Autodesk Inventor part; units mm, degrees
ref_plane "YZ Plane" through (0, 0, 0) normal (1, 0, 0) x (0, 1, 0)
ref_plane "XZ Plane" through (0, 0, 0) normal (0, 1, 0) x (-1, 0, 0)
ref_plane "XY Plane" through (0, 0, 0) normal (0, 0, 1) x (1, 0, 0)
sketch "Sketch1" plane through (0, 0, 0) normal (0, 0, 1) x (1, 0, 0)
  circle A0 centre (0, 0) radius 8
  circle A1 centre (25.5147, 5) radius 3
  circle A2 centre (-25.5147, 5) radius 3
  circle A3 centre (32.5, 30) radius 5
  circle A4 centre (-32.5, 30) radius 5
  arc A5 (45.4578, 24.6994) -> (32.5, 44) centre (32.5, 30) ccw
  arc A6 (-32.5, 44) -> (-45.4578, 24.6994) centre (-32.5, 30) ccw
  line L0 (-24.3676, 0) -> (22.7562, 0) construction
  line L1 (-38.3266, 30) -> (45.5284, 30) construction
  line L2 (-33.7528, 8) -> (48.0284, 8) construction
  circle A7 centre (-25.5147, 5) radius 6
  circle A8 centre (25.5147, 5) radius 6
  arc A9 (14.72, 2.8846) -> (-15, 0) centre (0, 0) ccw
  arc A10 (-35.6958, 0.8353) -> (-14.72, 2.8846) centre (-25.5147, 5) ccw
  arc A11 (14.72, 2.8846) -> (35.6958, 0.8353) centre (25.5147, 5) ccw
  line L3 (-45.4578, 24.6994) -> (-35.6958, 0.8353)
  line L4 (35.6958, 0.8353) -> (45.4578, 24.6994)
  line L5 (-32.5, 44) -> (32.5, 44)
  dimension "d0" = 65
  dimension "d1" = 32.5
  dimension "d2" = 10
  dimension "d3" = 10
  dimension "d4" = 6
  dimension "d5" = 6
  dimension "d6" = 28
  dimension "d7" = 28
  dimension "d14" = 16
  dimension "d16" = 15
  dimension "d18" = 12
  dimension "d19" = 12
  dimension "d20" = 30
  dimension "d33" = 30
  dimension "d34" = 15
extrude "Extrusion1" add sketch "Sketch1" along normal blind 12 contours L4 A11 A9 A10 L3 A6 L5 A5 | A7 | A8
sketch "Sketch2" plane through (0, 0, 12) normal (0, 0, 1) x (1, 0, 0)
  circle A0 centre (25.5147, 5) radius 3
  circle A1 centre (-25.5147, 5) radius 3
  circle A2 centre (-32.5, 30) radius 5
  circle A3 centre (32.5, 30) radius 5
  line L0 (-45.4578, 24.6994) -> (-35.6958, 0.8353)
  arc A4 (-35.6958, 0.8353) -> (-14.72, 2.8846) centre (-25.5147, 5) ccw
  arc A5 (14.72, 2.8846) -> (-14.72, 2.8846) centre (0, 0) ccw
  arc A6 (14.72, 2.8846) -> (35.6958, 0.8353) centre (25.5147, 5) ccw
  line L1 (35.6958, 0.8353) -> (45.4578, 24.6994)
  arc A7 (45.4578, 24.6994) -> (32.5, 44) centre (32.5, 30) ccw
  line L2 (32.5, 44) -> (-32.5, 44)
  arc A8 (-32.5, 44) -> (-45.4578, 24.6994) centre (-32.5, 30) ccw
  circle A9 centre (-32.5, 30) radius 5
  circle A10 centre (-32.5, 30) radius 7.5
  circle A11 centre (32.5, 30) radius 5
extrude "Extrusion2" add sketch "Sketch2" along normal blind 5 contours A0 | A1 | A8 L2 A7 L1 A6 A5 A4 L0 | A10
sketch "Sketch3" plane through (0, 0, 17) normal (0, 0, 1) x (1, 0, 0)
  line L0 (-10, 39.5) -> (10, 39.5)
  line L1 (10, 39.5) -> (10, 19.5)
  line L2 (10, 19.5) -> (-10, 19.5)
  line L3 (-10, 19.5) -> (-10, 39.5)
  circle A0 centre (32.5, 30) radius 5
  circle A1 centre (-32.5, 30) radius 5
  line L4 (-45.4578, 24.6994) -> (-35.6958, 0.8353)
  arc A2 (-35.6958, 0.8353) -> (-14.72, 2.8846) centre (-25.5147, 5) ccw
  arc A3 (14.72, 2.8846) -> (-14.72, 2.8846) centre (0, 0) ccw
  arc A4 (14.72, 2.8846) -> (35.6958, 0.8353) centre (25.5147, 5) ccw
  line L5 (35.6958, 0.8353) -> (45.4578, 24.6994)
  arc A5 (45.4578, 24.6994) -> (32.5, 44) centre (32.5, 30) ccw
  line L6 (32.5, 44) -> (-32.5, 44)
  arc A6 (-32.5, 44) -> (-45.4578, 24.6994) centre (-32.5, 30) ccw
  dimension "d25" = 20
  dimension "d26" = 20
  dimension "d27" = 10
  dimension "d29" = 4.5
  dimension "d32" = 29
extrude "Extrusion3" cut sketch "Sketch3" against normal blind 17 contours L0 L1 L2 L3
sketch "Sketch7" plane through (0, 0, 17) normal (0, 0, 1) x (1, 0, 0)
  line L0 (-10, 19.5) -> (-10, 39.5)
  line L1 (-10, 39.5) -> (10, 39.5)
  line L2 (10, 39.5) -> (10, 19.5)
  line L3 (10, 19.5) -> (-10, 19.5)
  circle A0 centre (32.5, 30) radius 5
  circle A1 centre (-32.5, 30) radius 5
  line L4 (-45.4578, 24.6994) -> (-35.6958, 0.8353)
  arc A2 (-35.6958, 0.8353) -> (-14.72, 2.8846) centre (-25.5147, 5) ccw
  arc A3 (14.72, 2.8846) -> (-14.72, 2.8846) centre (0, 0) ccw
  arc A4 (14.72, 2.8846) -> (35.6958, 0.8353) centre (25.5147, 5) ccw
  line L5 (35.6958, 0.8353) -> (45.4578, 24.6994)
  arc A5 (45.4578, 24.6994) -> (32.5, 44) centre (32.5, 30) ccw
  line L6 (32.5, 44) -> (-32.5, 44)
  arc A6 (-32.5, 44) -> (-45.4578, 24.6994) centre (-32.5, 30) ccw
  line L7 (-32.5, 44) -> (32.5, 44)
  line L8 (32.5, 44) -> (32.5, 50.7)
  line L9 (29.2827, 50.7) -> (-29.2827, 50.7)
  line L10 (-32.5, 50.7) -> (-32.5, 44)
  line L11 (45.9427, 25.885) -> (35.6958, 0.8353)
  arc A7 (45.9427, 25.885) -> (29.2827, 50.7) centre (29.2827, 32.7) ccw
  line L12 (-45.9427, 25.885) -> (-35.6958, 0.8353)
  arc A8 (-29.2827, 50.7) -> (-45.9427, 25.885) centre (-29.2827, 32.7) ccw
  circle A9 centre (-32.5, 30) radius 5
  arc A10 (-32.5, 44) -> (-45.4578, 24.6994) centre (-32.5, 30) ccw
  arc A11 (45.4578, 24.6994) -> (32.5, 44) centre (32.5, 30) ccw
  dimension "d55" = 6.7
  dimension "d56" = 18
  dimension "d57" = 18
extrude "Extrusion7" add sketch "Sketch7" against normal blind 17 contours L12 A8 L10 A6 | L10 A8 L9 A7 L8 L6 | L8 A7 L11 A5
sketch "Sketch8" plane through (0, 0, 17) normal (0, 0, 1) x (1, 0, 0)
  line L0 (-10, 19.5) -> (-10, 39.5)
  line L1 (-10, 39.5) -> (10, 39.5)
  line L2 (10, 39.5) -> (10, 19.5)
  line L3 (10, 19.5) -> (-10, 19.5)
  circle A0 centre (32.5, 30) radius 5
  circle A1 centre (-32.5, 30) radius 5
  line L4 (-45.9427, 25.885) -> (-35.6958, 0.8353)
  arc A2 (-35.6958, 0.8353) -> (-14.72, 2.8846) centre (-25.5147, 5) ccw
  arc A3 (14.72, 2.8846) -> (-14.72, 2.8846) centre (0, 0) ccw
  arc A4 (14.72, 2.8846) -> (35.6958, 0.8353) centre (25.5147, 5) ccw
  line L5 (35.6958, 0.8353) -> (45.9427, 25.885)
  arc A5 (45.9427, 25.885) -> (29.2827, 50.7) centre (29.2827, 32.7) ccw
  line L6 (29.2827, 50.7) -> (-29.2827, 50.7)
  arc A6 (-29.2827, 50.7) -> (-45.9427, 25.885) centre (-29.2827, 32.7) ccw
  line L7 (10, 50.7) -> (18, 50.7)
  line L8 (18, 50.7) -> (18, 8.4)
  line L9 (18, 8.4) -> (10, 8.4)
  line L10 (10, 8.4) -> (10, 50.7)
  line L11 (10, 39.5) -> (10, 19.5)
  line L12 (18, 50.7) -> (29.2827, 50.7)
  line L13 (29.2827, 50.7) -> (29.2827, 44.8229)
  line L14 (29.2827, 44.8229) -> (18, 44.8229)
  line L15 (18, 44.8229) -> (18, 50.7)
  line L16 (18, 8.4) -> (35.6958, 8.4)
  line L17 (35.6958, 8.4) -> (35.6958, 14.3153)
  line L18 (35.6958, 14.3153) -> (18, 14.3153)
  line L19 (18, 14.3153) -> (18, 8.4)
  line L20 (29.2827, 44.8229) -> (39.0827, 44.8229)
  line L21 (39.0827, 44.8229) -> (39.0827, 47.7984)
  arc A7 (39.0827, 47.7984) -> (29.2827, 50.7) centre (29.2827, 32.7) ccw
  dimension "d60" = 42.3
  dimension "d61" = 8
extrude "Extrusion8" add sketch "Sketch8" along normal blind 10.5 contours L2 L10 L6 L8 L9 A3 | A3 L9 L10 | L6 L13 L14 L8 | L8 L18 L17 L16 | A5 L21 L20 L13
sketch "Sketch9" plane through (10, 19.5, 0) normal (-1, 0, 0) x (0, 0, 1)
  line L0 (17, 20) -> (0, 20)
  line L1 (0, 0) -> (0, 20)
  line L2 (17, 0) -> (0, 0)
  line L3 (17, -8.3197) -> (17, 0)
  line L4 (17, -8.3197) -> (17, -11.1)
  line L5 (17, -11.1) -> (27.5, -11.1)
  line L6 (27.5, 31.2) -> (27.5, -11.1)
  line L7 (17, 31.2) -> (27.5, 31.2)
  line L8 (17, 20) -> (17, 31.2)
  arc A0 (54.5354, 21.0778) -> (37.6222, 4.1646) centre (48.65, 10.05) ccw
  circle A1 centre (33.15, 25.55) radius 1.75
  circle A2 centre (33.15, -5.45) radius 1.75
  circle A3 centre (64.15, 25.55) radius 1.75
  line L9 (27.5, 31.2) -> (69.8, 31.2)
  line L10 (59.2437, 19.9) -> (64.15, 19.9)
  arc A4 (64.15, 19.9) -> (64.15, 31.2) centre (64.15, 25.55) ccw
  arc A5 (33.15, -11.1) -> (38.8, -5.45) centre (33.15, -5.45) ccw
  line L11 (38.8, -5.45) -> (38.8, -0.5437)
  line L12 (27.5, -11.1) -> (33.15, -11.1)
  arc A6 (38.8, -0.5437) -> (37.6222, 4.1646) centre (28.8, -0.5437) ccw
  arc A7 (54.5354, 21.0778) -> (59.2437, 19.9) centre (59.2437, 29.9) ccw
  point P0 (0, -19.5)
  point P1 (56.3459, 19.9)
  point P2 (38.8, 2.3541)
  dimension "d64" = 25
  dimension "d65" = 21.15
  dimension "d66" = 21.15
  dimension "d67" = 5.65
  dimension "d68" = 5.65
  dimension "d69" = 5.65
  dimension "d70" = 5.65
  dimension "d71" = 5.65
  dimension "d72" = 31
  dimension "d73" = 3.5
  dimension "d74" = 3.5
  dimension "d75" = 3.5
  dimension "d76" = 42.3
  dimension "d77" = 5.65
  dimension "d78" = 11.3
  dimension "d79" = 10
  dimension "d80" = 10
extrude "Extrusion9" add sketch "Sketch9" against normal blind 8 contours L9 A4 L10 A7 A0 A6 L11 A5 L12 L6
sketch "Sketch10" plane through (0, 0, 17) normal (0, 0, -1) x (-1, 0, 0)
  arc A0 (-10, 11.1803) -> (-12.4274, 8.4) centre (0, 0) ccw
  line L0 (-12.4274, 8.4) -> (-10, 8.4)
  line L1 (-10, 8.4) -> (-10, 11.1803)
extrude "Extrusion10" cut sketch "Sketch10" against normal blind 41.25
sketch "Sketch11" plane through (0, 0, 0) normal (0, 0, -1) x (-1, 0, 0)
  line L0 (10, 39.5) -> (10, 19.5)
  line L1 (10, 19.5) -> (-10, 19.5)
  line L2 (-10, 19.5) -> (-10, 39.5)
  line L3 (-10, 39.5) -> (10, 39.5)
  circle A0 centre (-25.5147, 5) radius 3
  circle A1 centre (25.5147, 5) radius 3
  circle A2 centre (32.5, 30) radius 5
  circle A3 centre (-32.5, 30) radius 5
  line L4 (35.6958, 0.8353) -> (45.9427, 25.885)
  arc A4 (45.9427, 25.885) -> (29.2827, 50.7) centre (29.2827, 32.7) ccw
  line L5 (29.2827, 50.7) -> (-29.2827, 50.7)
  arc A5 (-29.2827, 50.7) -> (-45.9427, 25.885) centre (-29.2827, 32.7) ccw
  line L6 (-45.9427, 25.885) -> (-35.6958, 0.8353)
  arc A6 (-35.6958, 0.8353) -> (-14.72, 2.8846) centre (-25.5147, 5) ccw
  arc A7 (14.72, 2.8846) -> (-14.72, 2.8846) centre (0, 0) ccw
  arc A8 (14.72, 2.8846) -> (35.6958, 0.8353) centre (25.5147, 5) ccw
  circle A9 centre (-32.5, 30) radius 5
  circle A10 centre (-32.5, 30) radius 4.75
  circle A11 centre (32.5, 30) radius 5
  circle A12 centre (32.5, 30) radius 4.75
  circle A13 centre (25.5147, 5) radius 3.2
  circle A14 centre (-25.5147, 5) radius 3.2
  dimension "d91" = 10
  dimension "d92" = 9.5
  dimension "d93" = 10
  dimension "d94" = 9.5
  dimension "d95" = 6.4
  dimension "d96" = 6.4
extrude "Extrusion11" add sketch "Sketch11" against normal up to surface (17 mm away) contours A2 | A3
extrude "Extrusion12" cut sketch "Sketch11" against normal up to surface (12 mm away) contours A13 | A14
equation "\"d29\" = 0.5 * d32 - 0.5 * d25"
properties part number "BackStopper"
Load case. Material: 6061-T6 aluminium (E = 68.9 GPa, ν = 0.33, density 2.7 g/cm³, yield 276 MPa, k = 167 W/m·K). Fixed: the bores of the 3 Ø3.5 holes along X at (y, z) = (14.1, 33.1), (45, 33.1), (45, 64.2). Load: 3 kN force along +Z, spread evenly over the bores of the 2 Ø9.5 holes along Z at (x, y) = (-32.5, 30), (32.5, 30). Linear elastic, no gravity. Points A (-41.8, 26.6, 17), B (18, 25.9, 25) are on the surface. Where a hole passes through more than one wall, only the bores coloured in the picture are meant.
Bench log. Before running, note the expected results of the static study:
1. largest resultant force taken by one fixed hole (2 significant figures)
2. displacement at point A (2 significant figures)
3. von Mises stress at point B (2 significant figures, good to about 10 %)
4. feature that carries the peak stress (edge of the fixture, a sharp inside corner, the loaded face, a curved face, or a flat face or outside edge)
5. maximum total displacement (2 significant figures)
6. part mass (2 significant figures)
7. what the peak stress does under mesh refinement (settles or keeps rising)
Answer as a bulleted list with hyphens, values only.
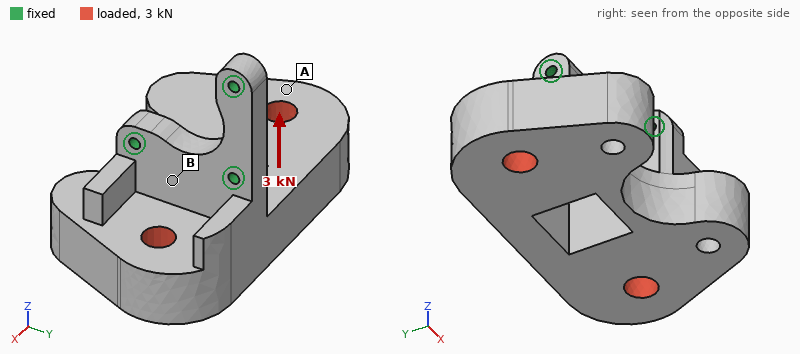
- 1.6 kN
- 0.48 mm
- 47 MPa
- edge of the fixture
- 0.56 mm
- 190 g
- keeps rising
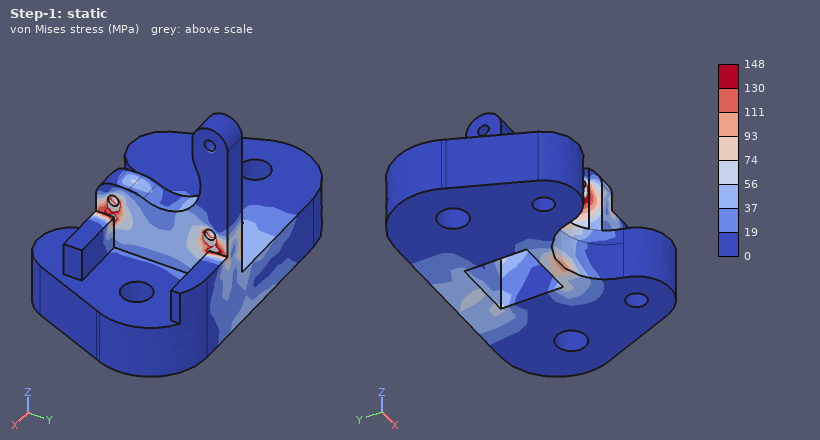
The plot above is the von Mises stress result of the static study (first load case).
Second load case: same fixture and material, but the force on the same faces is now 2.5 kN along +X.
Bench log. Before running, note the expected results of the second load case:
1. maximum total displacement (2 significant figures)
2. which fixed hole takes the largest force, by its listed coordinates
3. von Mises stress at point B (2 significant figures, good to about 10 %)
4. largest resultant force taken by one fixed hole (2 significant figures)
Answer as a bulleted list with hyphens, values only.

- 0.43 mm
- (45, 33.1)
- 50 MPa
- 1.5 kN
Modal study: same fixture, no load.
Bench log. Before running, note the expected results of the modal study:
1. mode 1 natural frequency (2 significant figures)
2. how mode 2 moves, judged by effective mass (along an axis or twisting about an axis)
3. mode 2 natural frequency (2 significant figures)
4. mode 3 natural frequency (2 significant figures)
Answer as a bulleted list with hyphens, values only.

- 890 Hz
- along Y
- 2000 Hz
- 3400 Hz
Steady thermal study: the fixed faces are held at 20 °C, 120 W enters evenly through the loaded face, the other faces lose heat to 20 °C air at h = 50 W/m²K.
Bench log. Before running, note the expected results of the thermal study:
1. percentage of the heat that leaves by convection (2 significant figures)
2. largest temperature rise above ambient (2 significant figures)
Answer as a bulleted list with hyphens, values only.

- 28 %
- 66 K
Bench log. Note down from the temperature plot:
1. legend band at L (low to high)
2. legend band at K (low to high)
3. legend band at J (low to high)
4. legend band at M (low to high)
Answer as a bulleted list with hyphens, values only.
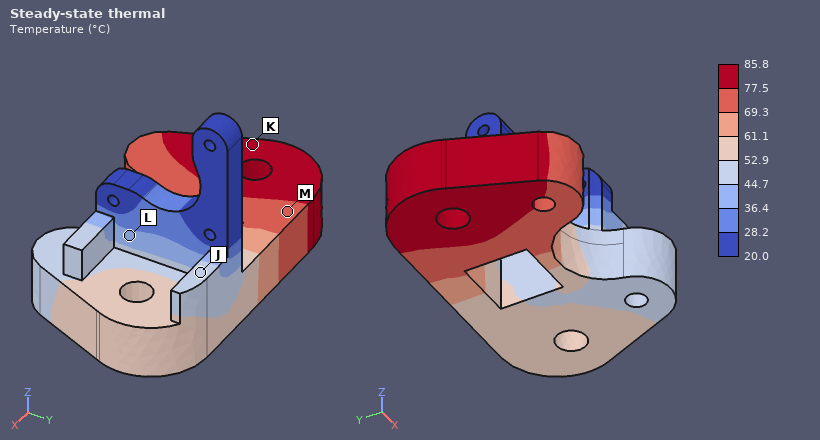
- 36.4 to 44.7 °C
- 77.5 to 85.8 °C
- 44.7 to 52.9 °C
- 69.3 to 77.5 °C
